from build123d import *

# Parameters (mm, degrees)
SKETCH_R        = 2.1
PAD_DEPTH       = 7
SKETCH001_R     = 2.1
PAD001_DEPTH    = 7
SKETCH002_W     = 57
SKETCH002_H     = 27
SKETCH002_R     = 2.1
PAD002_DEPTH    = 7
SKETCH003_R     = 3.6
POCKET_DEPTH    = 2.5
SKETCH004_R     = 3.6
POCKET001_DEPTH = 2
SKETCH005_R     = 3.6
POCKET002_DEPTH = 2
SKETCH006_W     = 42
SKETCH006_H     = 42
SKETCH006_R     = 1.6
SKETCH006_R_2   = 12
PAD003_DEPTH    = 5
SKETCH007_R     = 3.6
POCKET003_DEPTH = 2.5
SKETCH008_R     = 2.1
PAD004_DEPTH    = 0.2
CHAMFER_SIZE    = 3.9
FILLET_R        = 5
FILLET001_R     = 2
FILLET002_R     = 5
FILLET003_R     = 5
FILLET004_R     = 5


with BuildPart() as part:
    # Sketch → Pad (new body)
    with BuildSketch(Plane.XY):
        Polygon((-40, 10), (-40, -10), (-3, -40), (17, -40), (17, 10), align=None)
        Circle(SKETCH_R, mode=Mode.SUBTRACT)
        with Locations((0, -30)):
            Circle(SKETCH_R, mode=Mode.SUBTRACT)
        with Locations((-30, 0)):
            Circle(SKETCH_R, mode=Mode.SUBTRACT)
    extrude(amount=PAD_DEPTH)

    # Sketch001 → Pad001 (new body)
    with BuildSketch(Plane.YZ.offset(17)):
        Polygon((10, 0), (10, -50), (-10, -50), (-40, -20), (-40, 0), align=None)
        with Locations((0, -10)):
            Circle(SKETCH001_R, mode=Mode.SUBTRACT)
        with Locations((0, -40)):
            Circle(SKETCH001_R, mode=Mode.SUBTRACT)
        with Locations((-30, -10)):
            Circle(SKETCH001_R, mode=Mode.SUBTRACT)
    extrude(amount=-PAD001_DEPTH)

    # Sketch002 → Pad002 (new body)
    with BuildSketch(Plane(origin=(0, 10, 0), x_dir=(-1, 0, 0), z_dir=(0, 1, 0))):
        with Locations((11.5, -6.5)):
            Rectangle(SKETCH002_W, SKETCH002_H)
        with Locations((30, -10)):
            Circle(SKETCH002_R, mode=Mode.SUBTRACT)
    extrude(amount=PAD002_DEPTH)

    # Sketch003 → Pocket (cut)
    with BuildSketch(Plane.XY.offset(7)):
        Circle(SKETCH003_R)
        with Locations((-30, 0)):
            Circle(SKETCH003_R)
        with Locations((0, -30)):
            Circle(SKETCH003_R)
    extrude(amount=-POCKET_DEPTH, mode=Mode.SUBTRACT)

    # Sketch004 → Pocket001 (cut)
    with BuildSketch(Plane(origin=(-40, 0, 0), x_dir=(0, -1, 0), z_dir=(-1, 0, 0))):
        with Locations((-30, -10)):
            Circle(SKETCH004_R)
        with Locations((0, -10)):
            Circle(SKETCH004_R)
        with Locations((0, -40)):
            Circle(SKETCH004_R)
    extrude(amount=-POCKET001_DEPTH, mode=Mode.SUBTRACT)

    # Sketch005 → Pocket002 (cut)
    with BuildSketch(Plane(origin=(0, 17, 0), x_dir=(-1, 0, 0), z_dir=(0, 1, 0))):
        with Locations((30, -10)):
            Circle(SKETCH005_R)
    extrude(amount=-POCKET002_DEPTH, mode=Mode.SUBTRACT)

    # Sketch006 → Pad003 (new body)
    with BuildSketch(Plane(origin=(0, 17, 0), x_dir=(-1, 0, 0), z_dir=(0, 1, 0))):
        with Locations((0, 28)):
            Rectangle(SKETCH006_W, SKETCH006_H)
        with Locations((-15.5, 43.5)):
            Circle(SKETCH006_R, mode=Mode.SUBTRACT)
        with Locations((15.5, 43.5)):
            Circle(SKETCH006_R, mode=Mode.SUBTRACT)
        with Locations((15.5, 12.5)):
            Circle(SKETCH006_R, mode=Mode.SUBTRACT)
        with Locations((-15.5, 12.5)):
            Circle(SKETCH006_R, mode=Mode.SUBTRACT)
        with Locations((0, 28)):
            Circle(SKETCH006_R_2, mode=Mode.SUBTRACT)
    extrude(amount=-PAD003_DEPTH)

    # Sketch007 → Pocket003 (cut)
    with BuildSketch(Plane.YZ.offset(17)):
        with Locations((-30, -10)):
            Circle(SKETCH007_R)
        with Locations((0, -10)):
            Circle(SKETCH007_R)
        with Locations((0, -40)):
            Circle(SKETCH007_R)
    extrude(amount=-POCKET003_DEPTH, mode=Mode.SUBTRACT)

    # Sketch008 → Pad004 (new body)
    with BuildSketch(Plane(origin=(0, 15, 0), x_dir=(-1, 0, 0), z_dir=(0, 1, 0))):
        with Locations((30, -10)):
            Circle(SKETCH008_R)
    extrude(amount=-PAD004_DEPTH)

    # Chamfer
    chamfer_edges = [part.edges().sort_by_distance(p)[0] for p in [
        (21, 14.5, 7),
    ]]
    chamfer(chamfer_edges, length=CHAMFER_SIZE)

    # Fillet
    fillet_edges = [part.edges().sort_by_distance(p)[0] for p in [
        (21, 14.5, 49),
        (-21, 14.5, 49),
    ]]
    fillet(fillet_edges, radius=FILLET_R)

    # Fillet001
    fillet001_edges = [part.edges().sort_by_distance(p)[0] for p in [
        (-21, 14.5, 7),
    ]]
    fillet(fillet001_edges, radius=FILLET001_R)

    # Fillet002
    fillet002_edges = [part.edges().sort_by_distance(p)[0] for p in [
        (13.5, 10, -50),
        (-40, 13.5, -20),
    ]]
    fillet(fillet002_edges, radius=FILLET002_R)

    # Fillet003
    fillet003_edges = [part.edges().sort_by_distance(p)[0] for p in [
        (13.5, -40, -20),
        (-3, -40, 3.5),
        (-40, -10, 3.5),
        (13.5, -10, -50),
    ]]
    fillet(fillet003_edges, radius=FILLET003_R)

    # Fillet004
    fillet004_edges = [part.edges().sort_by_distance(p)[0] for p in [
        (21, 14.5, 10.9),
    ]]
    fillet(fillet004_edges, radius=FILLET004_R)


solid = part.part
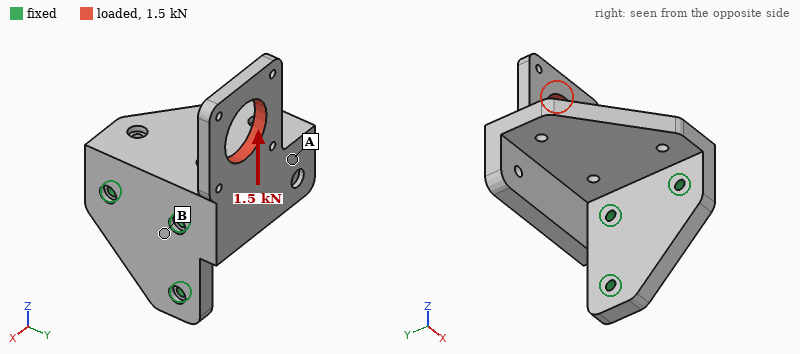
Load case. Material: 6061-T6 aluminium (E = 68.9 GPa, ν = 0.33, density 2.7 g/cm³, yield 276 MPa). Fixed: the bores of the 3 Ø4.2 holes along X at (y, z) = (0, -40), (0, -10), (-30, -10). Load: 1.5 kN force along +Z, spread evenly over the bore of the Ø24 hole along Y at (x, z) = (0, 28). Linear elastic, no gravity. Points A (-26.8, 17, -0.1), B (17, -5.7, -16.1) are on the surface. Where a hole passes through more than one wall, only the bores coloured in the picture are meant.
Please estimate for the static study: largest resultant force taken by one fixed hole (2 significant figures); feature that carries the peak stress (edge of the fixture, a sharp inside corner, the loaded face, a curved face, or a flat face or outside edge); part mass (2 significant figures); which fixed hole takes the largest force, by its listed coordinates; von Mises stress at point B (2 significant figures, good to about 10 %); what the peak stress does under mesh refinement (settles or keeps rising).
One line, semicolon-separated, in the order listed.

1.8 kN; edge of the fixture; 120 g; (0, -10); 18 MPa; keeps rising
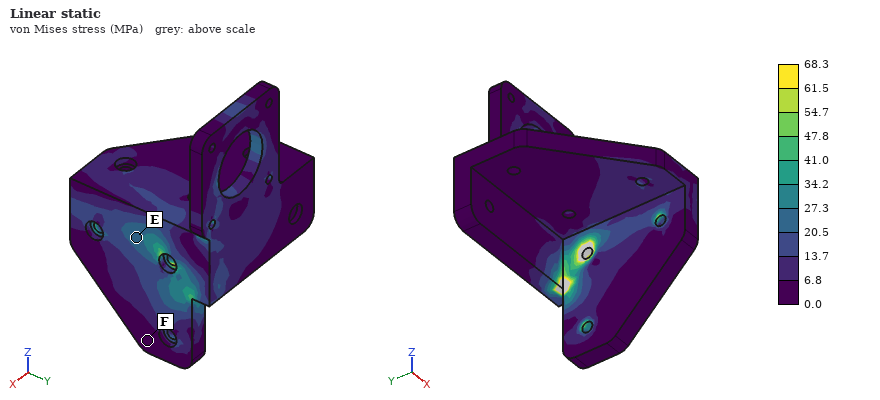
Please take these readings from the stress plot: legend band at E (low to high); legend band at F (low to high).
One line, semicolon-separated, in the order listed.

20.5 to 27.3 MPa; 0.0 to 6.8 MPa
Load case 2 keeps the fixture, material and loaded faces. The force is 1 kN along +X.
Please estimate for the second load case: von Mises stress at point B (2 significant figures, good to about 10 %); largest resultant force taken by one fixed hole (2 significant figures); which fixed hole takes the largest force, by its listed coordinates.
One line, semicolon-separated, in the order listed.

31 MPa; 2.3 kN; (0, -10)
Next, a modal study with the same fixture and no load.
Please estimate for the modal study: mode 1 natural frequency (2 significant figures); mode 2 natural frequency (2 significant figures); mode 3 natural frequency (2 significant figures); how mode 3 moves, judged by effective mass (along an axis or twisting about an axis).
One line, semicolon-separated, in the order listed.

1500 Hz; 1800 Hz; 3100 Hz; along Y
